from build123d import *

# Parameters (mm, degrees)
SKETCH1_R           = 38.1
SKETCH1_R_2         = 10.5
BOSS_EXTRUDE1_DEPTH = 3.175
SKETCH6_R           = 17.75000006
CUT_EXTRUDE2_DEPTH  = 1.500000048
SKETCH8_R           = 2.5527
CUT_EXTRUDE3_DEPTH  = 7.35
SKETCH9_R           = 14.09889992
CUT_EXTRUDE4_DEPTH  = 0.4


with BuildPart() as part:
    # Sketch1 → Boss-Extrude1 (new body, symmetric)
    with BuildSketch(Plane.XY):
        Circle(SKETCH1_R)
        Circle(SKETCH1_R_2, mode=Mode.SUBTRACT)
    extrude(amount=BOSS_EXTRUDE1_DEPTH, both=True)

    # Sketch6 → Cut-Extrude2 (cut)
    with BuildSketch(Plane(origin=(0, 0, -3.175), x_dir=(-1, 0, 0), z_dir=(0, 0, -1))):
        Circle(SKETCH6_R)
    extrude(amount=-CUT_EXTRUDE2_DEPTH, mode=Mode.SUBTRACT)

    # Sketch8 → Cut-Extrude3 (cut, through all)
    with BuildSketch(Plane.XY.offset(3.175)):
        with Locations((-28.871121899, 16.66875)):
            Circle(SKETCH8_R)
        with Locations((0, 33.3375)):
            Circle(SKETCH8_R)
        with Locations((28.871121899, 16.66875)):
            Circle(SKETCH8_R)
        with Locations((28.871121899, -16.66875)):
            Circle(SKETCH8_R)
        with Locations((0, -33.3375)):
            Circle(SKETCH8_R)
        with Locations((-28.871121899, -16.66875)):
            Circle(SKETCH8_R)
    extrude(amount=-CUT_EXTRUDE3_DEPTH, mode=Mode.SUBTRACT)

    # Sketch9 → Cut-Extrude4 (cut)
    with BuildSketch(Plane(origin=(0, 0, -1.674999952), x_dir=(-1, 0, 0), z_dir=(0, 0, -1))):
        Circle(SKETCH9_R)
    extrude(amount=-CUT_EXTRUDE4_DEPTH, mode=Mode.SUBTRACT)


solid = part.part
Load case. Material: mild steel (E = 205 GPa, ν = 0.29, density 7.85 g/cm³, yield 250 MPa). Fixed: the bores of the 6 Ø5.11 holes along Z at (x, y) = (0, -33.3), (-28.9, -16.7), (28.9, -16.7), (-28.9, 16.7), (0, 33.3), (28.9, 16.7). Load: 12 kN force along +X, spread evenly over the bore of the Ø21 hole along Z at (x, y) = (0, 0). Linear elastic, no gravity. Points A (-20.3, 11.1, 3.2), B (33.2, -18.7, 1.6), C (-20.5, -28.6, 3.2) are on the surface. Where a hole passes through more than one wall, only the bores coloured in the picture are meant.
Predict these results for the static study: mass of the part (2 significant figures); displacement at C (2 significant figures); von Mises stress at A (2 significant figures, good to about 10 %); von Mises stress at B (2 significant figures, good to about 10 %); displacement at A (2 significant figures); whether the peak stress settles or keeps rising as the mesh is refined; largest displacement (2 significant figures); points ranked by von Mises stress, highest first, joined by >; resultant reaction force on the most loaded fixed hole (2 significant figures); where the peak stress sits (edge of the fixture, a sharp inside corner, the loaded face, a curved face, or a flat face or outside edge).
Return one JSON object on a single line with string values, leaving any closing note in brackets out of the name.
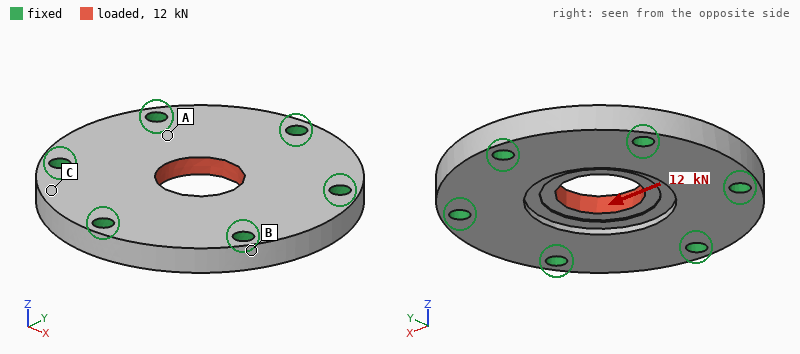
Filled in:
{"mass of the part": "200 g", "displacement at C": "1.0 µm", "von Mises stress at A": "37 MPa", "von Mises stress at B": "16 MPa", "displacement at A": "1.7 µm", "whether the peak stress settles or keeps rising as the mesh is refined": "keeps rising", "largest displacement": "4.8 µm", "points ranked by von Mises stress, highest first, joined by >": "A > B > C", "resultant reaction force on the most loaded fixed hole": "2.6 kN", "where the peak stress sits": "edge of the fixture"}
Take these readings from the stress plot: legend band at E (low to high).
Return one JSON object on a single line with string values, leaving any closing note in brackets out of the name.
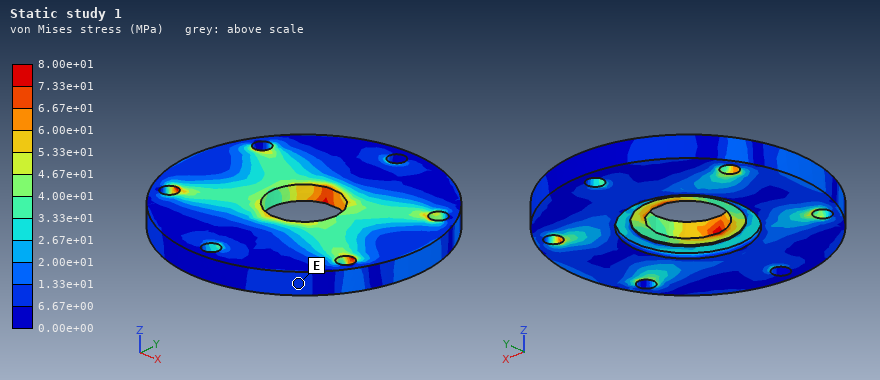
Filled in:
{"legend band at E": "6.67e+00 to 1.33e+01 MPa"}
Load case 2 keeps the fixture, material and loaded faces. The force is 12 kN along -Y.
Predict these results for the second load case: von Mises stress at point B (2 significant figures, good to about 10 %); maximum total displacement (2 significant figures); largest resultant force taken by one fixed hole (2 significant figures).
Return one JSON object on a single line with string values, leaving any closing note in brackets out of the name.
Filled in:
{"von Mises stress at point B": "8.4 MPa", "maximum total displacement": "4.7 µm", "largest resultant force taken by one fixed hole": "3.0 kN"}
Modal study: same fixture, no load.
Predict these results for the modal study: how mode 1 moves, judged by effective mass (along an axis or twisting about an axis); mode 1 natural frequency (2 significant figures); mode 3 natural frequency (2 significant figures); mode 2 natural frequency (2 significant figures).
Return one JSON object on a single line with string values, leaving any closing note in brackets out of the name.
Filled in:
{"how mode 1 moves, judged by effective mass": "along Z", "mode 1 natural frequency": "13 kHz", "mode 3 natural frequency": "19 kHz", "mode 2 natural frequency": "19 kHz"}
